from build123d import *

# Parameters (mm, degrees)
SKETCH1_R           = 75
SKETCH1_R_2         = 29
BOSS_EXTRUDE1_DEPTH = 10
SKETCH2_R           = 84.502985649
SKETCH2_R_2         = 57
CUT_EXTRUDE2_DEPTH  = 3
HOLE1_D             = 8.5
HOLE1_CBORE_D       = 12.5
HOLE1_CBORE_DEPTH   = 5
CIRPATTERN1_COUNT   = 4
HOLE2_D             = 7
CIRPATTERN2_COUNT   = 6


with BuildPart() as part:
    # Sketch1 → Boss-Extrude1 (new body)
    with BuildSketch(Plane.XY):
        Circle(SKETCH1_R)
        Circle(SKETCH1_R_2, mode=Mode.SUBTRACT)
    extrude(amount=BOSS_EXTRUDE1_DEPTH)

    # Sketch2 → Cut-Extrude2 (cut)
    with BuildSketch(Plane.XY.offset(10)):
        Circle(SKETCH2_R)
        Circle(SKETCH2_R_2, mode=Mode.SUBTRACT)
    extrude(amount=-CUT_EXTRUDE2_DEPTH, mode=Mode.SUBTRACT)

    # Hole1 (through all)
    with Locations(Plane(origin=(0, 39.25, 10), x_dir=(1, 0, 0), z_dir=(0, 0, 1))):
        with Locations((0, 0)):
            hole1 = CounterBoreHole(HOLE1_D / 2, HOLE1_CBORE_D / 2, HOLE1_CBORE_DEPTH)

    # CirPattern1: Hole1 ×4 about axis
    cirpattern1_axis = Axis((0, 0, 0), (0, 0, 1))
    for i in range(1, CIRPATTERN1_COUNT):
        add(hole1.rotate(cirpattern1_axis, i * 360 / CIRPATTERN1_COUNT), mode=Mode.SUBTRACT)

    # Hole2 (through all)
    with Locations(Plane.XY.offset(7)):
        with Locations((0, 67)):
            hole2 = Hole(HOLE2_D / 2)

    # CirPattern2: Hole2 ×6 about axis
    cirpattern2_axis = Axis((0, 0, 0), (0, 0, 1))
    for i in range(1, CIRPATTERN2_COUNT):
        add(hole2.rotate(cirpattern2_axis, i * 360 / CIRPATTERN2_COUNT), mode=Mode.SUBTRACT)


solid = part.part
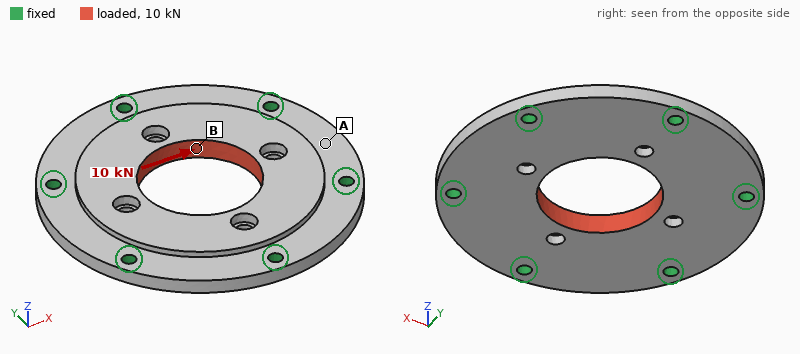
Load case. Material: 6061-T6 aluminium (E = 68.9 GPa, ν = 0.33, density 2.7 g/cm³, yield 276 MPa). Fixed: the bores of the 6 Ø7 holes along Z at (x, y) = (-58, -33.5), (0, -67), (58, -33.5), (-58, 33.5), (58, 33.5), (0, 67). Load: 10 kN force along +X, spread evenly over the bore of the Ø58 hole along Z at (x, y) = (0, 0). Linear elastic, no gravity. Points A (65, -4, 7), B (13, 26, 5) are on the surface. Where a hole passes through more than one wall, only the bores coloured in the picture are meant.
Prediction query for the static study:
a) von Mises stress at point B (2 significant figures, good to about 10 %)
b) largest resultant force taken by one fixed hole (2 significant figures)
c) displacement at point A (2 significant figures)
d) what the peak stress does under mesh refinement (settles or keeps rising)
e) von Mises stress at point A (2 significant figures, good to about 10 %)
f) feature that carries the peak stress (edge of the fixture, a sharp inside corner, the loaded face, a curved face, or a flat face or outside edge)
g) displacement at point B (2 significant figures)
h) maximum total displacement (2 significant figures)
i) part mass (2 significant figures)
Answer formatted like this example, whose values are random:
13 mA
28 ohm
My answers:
8.8 MPa
2.1 kN
4.7 µm
keeps rising
3.4 MPa
edge of the fixture
6.0 µm
9.4 µm
330 g
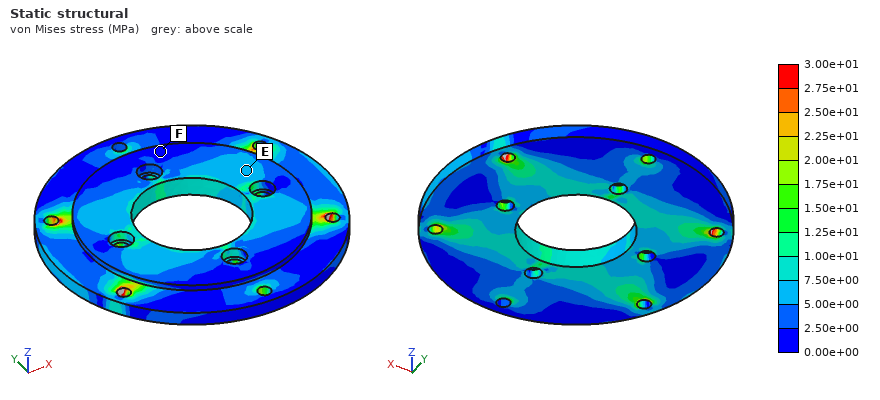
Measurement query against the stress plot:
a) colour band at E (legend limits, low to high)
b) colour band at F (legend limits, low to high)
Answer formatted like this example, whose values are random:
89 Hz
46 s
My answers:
5.00e+00 to 7.50e+00 MPa
0.00e+00 to 2.50e+00 MPa
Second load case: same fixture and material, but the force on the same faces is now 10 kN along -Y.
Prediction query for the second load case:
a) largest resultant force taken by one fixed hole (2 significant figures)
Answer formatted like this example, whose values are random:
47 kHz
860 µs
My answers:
2.3 kN
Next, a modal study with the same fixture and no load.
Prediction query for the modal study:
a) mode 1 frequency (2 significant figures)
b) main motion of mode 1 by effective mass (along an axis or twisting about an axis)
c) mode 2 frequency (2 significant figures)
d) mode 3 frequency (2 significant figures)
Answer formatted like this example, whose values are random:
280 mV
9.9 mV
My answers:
4300 Hz
along Z
6400 Hz
6500 Hz
